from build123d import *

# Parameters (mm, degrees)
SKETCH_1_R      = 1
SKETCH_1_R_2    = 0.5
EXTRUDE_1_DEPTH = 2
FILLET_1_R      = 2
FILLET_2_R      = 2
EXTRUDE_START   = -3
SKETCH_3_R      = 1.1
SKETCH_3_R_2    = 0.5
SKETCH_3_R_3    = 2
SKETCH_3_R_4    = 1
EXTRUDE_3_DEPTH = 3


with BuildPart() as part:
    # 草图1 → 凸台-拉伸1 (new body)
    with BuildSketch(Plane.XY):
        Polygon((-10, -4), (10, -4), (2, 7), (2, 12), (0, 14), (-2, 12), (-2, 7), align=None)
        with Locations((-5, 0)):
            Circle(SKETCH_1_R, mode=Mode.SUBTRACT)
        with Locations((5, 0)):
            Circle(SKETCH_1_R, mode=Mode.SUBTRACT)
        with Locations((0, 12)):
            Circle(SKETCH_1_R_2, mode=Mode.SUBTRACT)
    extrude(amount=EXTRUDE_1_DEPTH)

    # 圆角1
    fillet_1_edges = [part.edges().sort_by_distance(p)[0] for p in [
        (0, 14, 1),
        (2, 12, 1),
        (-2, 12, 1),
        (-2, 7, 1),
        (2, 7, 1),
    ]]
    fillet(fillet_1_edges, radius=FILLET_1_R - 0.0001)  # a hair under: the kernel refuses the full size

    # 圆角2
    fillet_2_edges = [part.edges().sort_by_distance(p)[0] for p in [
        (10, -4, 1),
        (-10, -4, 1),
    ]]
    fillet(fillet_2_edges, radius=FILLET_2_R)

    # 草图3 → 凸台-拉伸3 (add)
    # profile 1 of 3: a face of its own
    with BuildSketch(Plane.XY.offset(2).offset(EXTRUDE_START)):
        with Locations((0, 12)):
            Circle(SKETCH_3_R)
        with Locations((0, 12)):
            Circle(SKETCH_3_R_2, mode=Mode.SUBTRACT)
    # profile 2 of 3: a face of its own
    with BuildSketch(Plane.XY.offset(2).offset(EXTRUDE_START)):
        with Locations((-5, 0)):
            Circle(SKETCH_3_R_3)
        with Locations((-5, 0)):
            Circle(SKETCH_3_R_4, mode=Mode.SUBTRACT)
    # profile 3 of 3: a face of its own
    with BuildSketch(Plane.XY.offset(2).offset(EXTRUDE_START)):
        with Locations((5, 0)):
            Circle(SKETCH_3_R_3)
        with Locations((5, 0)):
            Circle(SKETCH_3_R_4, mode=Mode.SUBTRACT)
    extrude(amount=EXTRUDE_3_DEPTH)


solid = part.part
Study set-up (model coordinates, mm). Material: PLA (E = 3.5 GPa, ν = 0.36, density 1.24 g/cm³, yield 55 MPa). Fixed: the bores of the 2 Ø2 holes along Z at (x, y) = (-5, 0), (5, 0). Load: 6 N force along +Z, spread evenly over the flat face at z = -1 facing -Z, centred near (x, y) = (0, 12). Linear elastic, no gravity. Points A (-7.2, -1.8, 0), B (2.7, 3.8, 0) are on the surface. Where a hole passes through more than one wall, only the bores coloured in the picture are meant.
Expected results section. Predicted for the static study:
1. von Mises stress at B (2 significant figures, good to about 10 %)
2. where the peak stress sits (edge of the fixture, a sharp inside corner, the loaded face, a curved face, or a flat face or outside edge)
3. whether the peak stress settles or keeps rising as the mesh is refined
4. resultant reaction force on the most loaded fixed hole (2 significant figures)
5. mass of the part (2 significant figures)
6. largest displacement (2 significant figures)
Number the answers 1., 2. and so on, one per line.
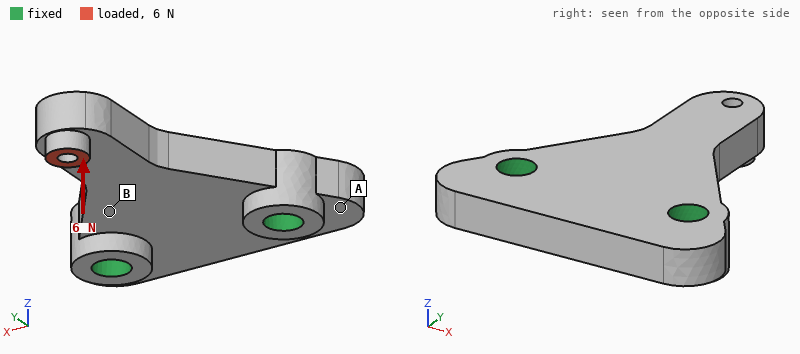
1. 9.6 MPa
2. edge of the fixture
3. keeps rising
4. 3.1 N
5. 0.38 g
6. 0.23 mm
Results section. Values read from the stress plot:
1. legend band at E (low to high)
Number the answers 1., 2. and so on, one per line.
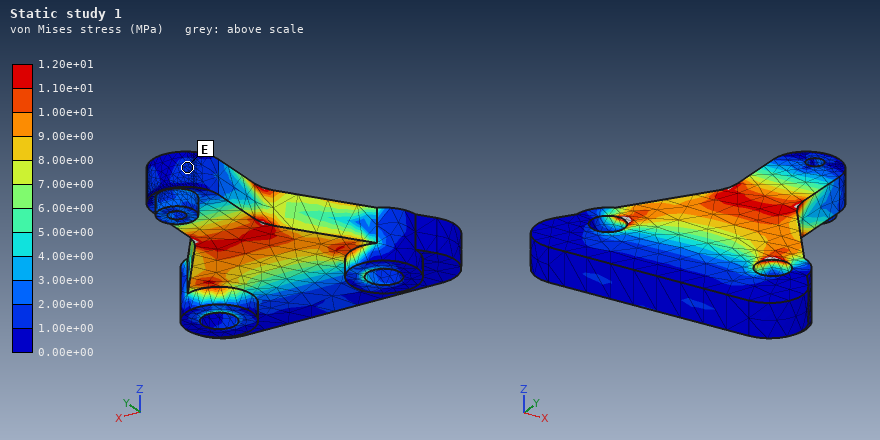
1. 1.00e+00 to 2.00e+00 MPa
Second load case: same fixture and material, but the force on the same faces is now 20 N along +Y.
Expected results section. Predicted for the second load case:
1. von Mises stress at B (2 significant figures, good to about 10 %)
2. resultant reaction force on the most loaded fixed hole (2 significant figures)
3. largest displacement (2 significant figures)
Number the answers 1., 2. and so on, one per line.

1. 8.9 MPa
2. 11 N
3. 0.26 mm
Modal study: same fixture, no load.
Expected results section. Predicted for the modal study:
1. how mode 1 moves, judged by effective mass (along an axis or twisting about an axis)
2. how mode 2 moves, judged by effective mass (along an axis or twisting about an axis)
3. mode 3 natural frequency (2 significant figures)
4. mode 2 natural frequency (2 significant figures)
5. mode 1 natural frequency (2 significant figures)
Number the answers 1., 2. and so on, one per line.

1. along Z
2. along X
3. 19 kHz
4. 15 kHz
5. 4600 Hz
